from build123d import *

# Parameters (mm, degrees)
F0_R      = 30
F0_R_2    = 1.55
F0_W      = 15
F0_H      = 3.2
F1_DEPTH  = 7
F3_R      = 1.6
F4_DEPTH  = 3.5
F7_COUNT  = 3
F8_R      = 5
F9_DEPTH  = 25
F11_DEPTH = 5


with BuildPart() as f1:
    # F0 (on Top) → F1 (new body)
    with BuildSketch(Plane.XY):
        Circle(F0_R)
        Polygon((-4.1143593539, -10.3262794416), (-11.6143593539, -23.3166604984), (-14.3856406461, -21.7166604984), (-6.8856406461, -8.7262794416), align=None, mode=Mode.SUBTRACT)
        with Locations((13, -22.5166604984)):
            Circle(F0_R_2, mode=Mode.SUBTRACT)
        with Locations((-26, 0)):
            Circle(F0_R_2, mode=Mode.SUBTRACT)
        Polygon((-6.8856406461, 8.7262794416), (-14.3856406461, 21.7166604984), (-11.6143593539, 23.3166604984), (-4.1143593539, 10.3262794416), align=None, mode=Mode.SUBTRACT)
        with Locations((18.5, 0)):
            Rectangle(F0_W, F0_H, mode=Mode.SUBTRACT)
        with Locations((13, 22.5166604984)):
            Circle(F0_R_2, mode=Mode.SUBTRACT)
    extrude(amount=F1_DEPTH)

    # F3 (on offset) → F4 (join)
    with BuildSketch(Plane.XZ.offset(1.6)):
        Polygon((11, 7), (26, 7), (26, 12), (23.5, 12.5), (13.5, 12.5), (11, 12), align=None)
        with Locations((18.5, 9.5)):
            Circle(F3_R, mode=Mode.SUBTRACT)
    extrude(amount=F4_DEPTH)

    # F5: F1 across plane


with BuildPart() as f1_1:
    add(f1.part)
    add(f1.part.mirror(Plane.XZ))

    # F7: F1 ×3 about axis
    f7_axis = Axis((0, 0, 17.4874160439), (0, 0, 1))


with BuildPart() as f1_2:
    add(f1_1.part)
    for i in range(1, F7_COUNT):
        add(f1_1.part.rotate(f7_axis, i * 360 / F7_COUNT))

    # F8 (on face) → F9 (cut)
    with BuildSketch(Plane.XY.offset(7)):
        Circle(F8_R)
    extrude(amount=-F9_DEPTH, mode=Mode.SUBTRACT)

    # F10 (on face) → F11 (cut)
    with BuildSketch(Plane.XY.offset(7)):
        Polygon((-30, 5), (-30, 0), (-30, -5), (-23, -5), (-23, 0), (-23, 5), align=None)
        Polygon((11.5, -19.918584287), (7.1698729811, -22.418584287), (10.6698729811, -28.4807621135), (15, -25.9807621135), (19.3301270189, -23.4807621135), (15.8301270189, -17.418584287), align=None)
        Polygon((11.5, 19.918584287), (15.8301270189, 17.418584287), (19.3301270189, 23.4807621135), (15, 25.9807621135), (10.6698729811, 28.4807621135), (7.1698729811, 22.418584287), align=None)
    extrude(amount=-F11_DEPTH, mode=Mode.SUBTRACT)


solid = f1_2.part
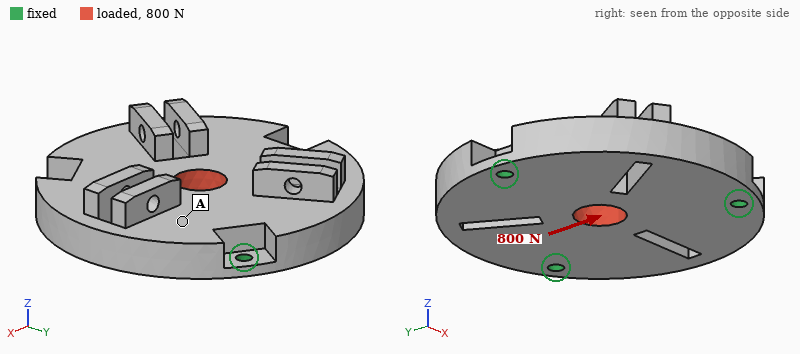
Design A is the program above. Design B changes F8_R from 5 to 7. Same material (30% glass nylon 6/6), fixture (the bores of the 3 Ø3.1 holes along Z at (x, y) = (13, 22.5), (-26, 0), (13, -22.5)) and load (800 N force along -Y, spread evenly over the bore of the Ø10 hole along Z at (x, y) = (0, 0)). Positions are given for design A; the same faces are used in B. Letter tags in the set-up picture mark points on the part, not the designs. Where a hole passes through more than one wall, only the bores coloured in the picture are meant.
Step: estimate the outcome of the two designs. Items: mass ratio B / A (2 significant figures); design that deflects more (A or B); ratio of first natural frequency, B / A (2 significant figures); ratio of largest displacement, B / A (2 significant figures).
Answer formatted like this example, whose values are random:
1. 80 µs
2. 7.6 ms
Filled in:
1. 0.97
2. B
3. 0.97
4. 1.1
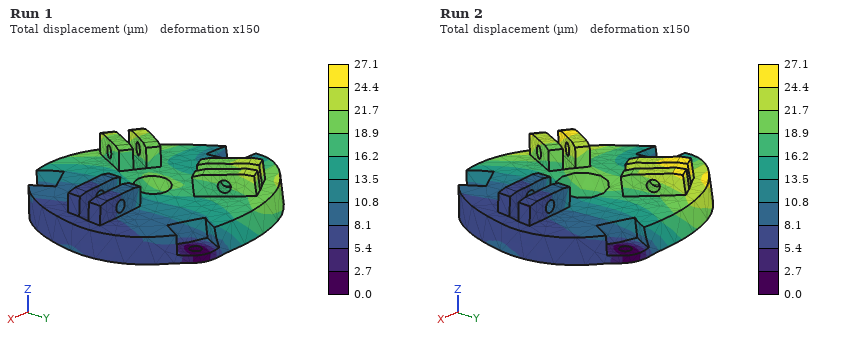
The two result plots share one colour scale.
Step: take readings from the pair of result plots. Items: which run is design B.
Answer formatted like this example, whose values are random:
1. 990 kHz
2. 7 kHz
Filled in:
1. Run 2
